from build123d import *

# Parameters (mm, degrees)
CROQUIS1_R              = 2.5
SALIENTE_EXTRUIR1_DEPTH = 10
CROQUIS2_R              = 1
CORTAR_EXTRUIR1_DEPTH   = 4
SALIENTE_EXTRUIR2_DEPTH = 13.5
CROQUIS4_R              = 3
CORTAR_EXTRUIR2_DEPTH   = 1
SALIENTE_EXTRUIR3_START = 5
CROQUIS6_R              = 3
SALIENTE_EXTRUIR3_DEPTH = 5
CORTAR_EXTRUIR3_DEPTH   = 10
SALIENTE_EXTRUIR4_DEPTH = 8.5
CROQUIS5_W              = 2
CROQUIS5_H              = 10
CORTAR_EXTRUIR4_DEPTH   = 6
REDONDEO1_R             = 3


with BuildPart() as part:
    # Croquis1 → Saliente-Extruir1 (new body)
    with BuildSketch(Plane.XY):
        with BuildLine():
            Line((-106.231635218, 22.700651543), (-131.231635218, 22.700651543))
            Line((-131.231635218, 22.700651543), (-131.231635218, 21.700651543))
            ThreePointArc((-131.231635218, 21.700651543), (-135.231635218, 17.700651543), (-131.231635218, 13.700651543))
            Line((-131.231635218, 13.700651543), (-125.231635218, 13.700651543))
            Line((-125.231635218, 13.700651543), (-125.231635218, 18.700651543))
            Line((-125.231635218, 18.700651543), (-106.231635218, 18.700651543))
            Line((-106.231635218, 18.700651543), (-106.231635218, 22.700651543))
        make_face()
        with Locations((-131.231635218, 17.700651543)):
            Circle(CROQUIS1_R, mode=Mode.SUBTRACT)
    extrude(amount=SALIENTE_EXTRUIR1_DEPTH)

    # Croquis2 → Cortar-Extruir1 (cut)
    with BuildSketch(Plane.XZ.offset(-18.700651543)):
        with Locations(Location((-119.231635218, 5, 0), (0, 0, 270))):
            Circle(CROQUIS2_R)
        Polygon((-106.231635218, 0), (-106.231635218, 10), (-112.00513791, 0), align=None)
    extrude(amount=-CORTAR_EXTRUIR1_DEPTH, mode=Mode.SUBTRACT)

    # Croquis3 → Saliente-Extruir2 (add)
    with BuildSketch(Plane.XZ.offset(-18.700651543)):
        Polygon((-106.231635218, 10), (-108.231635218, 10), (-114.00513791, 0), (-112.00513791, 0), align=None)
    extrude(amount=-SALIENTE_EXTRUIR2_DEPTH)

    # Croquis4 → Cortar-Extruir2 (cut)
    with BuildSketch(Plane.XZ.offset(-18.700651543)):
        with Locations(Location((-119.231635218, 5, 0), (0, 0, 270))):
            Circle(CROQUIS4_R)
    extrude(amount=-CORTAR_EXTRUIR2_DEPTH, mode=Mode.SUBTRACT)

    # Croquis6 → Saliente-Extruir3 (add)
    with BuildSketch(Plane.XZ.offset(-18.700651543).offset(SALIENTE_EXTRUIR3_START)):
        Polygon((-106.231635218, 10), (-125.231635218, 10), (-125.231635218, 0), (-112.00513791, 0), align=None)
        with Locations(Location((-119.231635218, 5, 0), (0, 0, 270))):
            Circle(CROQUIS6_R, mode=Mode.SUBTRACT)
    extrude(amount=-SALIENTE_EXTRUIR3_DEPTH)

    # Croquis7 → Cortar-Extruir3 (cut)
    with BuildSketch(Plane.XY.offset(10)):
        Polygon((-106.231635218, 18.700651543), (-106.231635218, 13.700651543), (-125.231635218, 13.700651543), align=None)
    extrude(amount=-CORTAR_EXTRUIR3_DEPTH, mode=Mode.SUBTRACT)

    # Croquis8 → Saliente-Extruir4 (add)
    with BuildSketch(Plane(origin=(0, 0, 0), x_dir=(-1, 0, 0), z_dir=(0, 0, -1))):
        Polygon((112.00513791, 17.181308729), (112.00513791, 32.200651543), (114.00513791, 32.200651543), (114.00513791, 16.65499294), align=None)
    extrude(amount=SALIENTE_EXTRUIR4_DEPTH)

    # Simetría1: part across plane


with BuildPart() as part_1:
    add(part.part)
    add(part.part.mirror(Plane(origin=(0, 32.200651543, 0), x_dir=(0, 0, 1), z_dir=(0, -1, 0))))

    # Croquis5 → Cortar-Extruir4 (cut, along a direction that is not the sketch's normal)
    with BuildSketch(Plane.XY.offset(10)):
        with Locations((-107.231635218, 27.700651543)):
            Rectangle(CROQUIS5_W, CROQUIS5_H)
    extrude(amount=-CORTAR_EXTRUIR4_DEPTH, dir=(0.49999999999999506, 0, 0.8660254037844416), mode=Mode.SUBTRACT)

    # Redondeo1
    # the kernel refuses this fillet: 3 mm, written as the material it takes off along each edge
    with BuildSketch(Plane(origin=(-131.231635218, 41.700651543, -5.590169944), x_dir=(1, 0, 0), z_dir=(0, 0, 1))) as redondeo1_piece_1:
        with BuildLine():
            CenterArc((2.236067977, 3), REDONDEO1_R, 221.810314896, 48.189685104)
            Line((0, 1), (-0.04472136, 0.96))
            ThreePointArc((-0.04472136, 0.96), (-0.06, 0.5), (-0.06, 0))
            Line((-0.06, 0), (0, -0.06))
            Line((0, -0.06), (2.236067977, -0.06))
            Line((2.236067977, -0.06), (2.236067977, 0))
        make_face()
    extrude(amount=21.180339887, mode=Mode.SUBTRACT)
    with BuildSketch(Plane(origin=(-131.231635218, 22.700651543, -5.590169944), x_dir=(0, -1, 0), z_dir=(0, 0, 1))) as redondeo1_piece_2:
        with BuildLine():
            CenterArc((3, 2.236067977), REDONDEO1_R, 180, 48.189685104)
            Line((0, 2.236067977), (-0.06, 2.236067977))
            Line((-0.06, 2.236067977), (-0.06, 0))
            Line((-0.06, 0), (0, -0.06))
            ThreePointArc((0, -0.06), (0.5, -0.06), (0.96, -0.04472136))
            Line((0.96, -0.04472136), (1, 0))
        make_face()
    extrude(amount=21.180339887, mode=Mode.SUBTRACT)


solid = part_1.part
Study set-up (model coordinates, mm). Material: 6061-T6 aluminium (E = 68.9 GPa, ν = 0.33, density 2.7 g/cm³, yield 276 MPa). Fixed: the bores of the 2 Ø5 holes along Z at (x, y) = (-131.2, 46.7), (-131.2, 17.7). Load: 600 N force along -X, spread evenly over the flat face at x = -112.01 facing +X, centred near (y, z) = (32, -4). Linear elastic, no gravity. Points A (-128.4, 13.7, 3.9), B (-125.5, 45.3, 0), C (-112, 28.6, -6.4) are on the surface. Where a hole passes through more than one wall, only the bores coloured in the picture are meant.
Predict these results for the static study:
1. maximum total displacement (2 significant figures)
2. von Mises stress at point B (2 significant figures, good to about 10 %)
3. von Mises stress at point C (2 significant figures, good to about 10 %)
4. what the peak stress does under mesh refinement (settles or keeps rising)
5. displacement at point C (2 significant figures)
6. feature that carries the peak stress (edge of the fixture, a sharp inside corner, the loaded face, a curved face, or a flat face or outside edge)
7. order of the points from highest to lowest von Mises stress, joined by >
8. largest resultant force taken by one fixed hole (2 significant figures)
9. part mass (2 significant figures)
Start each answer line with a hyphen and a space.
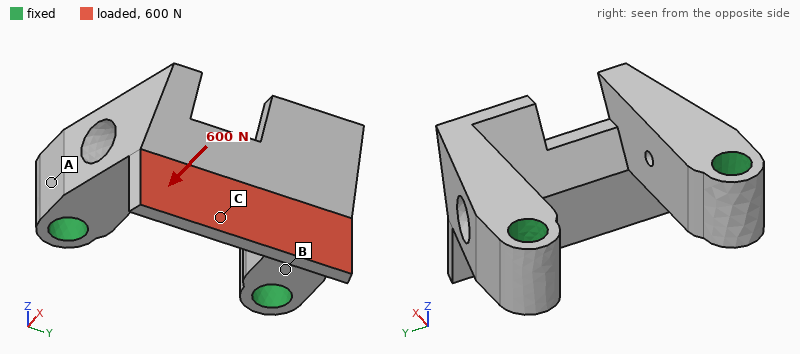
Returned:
- 0.13 mm
- 29 MPa
- 50 MPa
- keeps rising
- 0.097 mm
- a sharp inside corner
- C > B > A
- 310 N
- 11 g
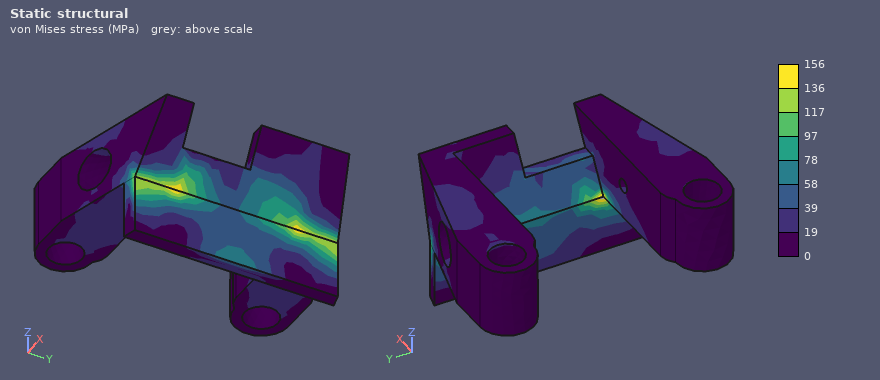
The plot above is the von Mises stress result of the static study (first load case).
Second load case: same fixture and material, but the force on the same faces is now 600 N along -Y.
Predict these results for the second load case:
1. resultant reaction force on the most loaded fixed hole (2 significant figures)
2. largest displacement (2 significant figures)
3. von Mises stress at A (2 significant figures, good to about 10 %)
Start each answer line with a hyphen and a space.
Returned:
- 340 N
- 39 µm
- 27 MPa
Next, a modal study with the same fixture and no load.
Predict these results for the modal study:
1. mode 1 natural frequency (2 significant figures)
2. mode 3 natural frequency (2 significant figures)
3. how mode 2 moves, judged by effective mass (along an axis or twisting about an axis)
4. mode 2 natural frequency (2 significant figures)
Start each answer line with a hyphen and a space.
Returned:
- 11 kHz
- 15 kHz
- along Y
- 12 kHz
